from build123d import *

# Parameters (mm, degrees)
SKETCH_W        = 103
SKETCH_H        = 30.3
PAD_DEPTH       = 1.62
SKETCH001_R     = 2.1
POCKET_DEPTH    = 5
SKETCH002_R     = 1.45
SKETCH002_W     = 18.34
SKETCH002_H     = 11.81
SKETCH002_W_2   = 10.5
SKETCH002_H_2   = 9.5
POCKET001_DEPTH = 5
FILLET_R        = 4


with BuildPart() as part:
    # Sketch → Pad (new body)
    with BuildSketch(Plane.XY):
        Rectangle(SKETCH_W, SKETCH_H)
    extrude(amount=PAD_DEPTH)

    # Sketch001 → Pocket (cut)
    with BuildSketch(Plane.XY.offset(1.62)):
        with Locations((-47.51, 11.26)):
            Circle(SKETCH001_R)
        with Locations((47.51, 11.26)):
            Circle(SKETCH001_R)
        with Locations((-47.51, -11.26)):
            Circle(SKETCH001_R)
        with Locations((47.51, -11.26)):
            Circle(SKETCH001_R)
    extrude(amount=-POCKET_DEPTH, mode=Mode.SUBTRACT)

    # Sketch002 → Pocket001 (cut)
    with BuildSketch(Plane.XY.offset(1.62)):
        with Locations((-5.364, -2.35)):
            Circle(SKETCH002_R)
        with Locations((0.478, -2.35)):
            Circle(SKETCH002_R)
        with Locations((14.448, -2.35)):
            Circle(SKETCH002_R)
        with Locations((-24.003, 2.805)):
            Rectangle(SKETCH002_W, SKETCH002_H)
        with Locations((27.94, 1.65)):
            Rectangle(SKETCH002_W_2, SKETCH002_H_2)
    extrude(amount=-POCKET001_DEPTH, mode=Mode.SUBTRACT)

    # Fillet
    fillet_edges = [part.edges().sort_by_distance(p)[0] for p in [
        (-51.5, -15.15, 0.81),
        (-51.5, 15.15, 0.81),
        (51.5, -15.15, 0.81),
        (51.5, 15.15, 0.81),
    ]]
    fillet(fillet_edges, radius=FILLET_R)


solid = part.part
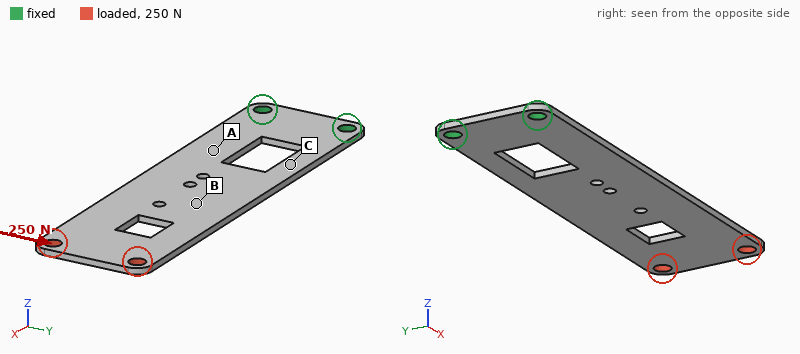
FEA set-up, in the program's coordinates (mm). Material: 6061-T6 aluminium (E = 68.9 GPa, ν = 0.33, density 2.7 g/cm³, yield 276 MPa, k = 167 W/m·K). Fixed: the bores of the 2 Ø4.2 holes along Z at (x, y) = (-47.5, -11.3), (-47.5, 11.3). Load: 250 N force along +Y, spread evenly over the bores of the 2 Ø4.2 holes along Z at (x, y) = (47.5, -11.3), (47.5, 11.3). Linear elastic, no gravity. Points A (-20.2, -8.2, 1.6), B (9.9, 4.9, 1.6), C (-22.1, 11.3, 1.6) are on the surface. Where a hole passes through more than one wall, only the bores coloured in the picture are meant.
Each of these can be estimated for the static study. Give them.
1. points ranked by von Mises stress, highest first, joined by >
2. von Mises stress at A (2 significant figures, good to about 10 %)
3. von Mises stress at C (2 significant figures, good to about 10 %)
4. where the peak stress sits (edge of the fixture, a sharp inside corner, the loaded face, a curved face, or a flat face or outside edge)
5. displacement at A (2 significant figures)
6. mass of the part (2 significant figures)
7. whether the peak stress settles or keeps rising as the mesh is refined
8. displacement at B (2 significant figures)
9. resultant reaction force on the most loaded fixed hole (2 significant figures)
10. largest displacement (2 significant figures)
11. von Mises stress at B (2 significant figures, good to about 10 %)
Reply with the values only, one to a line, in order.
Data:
C > A > B
44 MPa
77 MPa
a sharp inside corner
0.059 mm
12 g
keeps rising
0.17 mm
1.0 kN
0.38 mm
17 MPa
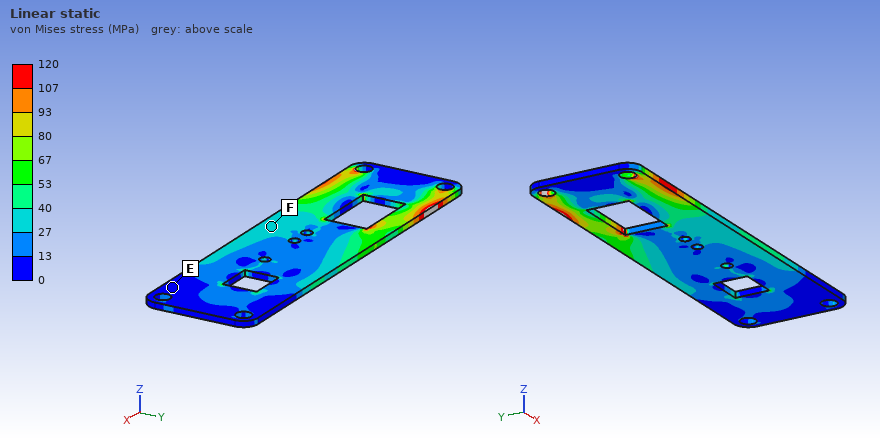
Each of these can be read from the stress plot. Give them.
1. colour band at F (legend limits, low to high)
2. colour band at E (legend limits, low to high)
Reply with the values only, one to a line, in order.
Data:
27 to 40 MPa
0 to 13 MPa
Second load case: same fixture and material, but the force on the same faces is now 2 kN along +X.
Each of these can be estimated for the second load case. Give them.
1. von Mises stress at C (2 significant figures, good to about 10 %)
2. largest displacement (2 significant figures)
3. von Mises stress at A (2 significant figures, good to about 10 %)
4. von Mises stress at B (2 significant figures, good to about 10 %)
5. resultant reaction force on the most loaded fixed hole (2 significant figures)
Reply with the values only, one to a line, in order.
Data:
84 MPa
0.11 mm
60 MPa
35 MPa
1.0 kN
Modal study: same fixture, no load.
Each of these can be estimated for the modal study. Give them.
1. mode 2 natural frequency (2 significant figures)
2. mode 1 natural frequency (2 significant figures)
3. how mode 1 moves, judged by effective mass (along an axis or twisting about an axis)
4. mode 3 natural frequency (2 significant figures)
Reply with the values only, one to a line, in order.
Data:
830 Hz
130 Hz
along Z
850 Hz
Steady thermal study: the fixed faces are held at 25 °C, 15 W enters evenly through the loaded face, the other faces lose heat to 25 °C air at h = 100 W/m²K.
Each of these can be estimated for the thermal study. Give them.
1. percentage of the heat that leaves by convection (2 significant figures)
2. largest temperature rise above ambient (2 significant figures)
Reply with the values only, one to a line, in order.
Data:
90 %
75 K
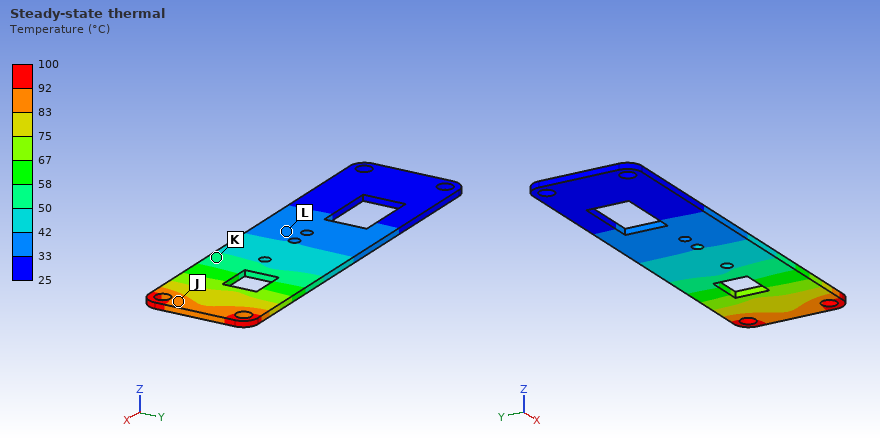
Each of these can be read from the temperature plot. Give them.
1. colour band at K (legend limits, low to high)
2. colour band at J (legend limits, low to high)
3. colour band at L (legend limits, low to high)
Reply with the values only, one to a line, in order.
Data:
50 to 58 °C
83 to 92 °C
33 to 42 °C
